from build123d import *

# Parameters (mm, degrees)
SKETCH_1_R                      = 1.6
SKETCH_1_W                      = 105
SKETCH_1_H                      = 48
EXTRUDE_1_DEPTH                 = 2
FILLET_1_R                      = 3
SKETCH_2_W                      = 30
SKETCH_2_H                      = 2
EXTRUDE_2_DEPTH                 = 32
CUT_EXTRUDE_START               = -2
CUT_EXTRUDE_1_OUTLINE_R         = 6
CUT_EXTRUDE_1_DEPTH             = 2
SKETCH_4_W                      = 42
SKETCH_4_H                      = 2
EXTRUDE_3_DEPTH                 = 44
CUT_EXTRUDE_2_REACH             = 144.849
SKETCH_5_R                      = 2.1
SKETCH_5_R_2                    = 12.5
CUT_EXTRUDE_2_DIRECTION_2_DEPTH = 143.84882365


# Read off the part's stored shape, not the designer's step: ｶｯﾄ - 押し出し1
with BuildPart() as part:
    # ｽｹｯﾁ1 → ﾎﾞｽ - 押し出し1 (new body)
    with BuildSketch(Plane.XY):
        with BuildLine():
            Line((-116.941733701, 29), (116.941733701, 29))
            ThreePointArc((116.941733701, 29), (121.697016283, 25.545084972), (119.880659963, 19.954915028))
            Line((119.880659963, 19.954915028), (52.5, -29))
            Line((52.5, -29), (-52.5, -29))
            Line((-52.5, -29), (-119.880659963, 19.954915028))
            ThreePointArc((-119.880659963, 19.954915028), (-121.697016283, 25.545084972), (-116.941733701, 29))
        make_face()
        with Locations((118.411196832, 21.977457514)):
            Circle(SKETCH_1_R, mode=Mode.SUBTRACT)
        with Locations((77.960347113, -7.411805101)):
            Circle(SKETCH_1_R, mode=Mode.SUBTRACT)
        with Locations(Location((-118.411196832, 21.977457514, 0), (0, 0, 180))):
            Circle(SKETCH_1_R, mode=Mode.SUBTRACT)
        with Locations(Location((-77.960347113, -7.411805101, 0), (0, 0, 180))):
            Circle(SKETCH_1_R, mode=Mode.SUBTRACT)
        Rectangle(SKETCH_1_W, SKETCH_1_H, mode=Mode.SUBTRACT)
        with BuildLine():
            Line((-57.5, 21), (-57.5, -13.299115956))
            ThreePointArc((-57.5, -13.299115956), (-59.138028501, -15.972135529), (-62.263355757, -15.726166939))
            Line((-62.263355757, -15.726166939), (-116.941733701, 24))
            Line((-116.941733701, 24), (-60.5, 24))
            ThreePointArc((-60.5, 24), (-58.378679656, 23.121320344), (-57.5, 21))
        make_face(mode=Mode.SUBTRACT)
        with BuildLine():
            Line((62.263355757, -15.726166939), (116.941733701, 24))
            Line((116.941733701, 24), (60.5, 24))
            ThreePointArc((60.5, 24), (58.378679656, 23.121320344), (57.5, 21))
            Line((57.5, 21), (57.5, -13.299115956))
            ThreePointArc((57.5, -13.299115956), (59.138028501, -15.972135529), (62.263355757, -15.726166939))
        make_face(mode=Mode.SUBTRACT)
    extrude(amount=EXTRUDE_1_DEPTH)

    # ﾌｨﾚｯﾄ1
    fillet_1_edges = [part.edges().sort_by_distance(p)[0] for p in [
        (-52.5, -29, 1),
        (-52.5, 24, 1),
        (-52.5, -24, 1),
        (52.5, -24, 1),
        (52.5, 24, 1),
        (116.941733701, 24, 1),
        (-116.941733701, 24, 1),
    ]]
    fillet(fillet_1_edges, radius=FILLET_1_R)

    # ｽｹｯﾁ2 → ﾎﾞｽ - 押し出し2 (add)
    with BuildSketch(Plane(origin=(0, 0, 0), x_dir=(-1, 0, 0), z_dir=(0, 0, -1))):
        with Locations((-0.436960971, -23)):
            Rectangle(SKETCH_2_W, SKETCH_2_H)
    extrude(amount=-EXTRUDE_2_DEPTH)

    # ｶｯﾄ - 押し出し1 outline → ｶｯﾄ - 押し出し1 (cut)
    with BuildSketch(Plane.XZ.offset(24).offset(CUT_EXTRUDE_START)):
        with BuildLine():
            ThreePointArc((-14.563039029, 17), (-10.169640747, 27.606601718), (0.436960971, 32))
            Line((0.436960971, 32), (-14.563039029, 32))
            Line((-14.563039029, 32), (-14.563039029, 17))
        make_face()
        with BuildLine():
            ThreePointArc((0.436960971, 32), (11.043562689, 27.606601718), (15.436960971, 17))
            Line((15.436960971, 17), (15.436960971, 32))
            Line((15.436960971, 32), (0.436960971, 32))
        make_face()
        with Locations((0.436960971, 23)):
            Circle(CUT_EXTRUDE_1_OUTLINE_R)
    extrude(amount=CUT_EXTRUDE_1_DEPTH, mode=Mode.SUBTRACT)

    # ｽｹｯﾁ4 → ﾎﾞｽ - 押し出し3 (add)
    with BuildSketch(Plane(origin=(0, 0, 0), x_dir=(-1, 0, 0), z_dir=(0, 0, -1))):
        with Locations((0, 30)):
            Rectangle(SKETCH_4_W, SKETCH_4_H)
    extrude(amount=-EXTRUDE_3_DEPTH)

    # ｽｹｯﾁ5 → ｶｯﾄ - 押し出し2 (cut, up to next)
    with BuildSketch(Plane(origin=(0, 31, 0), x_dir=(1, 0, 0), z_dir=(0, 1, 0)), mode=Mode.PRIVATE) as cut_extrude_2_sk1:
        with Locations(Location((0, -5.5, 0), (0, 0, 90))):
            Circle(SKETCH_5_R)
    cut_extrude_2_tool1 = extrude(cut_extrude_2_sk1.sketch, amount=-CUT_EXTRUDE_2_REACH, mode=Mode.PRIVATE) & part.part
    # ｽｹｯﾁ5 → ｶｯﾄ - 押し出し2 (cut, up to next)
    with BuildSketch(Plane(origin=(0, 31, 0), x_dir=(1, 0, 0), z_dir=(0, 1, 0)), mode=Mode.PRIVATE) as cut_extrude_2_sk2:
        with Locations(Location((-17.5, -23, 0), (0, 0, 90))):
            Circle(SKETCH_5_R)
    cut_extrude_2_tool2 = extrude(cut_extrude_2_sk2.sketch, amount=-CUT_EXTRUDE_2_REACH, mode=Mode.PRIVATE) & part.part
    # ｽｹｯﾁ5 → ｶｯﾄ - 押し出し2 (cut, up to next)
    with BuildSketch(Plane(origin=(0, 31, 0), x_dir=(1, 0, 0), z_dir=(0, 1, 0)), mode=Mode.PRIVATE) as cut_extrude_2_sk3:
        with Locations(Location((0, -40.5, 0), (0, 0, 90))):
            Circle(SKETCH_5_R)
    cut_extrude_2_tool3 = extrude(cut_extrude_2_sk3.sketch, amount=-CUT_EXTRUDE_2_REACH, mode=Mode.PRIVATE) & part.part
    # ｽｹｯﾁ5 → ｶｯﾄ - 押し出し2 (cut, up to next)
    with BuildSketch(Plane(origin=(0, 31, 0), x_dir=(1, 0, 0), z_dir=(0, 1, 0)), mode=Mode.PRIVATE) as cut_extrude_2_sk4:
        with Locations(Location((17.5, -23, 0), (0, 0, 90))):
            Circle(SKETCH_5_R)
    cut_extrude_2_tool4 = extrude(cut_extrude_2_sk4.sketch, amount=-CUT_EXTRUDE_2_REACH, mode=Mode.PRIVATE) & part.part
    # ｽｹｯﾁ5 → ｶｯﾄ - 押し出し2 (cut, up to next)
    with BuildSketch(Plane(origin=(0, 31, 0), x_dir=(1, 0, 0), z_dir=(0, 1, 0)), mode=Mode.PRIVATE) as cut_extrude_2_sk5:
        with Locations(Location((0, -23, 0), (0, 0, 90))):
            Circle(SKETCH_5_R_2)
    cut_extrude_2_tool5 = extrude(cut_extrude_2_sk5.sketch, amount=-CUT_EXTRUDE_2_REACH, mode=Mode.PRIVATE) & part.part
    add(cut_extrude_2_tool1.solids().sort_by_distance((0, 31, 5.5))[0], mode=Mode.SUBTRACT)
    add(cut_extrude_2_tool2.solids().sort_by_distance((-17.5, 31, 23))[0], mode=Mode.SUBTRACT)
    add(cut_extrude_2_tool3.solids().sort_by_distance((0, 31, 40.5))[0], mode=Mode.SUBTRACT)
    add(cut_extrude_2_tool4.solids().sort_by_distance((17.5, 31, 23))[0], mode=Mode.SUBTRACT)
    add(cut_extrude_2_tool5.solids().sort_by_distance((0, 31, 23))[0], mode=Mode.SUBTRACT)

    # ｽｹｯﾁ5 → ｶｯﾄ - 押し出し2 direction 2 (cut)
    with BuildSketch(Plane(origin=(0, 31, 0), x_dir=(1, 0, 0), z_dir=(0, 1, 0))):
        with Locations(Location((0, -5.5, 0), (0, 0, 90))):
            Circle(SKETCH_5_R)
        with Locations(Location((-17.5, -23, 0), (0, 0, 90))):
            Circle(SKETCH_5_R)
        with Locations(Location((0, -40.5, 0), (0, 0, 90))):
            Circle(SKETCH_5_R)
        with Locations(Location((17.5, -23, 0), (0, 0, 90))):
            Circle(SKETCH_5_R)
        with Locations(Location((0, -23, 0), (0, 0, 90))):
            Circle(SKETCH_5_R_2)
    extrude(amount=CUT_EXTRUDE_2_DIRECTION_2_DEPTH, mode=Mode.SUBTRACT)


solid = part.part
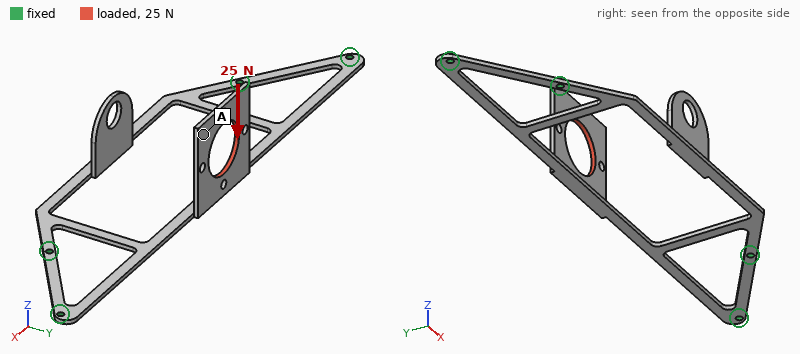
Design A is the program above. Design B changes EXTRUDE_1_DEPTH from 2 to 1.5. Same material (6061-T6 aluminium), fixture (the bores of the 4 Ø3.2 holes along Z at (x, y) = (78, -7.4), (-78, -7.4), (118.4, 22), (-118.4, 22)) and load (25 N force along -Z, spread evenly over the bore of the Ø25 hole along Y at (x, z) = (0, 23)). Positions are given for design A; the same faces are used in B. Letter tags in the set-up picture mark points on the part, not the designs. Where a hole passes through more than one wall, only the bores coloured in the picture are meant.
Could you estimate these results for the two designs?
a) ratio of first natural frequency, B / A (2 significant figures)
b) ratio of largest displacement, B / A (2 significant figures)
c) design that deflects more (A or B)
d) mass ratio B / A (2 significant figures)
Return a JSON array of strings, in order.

["0.69", "2.3", "B", "0.85"]
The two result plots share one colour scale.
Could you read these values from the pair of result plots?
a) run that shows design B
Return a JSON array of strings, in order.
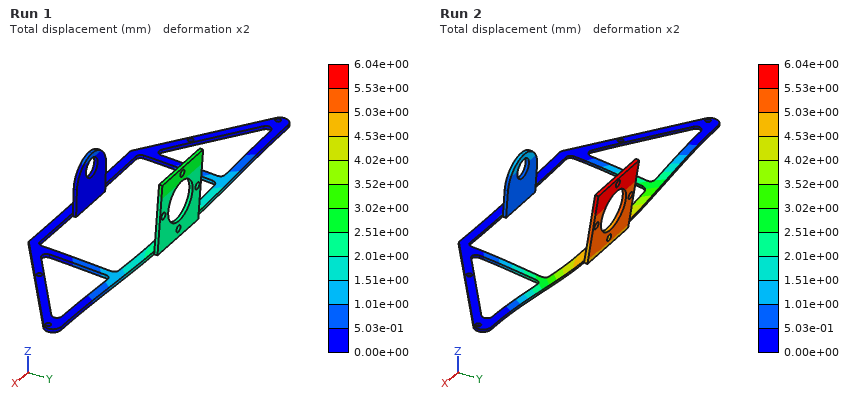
["Run 2"]
